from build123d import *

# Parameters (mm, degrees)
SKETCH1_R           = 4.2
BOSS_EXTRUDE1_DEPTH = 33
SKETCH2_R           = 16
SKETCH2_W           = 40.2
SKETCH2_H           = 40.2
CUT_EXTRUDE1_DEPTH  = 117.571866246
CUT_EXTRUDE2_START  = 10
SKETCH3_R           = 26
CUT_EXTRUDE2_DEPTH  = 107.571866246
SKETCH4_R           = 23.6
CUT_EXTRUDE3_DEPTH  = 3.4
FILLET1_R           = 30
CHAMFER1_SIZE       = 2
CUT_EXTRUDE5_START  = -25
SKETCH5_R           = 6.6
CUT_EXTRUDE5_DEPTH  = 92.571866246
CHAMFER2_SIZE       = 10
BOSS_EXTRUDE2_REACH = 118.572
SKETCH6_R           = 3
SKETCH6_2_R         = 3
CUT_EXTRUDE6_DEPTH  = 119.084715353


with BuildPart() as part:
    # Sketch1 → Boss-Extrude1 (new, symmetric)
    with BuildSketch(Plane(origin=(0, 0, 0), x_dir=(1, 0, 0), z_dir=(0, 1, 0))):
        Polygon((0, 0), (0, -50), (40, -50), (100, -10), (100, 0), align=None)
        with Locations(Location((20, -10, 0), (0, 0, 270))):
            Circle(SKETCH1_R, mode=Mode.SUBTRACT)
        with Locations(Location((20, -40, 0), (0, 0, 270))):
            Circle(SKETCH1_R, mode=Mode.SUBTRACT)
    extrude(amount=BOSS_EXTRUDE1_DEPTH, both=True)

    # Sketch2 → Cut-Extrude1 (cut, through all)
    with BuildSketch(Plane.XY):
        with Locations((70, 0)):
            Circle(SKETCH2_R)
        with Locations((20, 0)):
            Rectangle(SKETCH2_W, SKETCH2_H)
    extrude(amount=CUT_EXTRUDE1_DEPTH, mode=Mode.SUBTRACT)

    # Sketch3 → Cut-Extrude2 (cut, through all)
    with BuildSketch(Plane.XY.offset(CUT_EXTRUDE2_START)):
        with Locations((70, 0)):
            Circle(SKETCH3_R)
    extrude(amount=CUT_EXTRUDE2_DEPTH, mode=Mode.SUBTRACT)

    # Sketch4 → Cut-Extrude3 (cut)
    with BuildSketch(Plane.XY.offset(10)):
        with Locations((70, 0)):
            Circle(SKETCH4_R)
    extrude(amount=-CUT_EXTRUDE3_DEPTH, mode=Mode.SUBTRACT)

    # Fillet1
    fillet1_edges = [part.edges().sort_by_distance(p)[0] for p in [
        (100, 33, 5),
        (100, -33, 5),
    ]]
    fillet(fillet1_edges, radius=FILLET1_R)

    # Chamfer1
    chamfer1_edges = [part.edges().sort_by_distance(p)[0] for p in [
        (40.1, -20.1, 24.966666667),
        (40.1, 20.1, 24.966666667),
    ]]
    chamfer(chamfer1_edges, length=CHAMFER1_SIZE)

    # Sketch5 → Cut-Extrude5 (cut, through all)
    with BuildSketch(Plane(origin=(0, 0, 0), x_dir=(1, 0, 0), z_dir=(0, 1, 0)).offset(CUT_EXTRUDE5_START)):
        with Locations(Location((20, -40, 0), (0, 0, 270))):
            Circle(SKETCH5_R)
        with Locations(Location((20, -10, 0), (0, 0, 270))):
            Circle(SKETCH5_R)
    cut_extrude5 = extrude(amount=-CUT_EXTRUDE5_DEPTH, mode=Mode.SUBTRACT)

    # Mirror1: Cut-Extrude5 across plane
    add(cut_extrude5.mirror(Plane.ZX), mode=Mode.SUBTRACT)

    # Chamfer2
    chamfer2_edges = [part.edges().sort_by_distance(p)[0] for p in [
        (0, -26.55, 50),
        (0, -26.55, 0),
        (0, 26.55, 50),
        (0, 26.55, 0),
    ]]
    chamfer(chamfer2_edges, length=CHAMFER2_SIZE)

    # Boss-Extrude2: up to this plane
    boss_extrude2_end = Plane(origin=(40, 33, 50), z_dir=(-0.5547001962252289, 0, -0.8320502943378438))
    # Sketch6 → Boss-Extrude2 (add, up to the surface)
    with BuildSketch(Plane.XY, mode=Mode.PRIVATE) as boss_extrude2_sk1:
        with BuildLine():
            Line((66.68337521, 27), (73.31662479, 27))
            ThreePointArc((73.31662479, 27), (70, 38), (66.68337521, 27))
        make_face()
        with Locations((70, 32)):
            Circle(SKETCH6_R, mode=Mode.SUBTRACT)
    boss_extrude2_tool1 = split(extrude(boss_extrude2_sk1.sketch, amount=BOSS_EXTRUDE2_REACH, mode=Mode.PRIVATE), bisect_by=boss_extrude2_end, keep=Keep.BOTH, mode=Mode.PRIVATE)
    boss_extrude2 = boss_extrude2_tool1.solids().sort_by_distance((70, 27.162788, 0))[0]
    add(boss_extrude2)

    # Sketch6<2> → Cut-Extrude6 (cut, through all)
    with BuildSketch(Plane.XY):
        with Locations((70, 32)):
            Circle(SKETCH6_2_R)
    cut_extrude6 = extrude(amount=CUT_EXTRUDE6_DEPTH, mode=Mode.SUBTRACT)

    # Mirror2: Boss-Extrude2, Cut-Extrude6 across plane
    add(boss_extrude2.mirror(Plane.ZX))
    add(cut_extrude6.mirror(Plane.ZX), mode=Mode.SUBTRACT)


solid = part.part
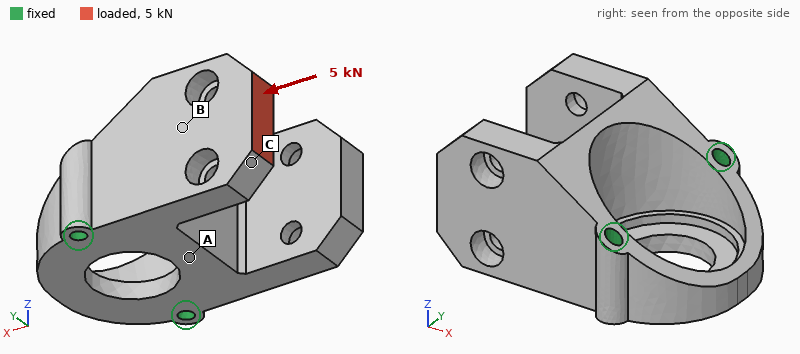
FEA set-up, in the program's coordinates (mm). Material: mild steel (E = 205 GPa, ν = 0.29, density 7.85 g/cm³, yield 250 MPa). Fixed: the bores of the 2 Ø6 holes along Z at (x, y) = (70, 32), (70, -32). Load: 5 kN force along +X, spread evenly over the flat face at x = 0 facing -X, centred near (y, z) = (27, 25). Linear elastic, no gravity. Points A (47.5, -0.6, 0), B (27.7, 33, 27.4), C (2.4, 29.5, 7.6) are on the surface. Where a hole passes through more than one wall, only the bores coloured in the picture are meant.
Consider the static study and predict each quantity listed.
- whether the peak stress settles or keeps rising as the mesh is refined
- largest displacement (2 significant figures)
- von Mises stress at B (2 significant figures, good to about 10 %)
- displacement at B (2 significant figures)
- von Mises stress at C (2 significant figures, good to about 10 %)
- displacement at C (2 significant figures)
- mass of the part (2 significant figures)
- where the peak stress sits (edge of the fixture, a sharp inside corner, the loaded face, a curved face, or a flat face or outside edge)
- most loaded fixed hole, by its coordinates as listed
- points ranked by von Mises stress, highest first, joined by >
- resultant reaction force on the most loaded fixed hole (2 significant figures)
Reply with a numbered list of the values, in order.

1. keeps rising
2. 12 µm
3. 17 MPa
4. 6.8 µm
5. 7.5 MPa
6. 8.9 µm
7. 820 g
8. edge of the fixture
9. (70, 32)
10. B > C > A
11. 4.8 kN
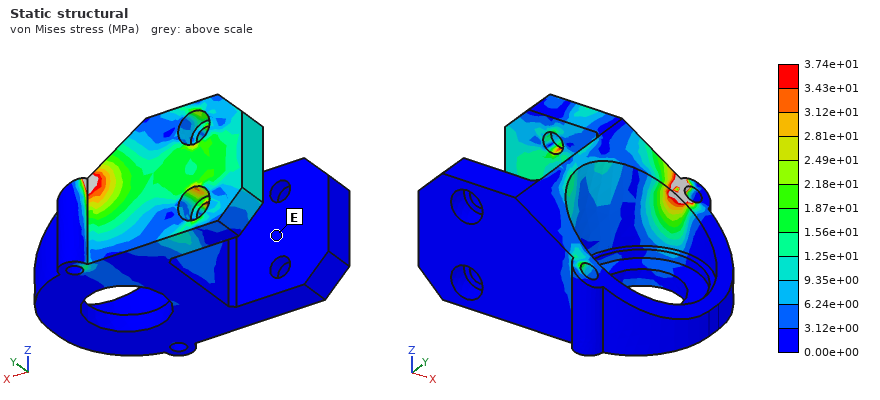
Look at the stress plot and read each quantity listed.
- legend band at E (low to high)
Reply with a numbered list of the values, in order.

1. 0.00e+00 to 3.12e+00 MPa
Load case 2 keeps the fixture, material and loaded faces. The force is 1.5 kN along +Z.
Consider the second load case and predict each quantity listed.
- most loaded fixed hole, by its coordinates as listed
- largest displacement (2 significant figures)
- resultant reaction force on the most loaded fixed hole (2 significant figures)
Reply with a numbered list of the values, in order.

1. (70, 32)
2. 24 µm
3. 1.4 kN
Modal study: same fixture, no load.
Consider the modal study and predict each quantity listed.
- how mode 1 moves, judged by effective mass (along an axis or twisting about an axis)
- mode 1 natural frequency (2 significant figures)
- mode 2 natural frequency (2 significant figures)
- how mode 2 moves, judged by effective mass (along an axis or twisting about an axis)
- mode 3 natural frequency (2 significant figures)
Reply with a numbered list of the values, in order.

1. along Y
2. 3100 Hz
3. 4000 Hz
4. along Z
5. 4200 Hz
